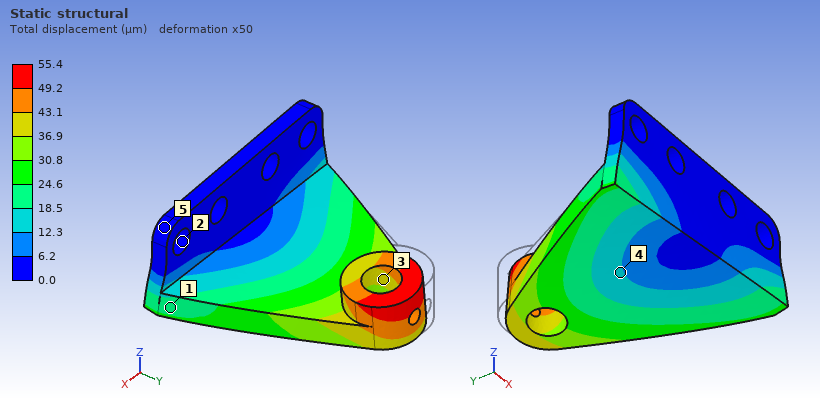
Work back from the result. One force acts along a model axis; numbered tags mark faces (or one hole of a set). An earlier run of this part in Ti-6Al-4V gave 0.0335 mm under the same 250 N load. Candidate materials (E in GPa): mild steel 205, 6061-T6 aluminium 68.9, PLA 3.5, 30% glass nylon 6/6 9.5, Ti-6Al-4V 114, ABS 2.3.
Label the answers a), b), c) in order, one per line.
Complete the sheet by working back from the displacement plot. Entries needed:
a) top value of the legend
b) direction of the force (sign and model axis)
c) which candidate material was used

a) 55.4 µm
b) +X
c) 6061-T6 aluminium
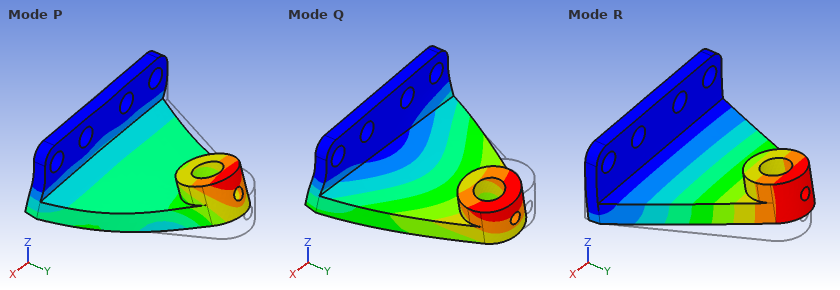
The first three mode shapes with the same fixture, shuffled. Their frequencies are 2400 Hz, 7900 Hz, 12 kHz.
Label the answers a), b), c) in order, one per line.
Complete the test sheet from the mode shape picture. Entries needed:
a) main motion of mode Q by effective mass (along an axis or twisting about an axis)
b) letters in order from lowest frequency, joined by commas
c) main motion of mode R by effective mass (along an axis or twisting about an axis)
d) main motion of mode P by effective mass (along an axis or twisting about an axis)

a) along X
b) R, Q, P
c) along Z
d) along Y
